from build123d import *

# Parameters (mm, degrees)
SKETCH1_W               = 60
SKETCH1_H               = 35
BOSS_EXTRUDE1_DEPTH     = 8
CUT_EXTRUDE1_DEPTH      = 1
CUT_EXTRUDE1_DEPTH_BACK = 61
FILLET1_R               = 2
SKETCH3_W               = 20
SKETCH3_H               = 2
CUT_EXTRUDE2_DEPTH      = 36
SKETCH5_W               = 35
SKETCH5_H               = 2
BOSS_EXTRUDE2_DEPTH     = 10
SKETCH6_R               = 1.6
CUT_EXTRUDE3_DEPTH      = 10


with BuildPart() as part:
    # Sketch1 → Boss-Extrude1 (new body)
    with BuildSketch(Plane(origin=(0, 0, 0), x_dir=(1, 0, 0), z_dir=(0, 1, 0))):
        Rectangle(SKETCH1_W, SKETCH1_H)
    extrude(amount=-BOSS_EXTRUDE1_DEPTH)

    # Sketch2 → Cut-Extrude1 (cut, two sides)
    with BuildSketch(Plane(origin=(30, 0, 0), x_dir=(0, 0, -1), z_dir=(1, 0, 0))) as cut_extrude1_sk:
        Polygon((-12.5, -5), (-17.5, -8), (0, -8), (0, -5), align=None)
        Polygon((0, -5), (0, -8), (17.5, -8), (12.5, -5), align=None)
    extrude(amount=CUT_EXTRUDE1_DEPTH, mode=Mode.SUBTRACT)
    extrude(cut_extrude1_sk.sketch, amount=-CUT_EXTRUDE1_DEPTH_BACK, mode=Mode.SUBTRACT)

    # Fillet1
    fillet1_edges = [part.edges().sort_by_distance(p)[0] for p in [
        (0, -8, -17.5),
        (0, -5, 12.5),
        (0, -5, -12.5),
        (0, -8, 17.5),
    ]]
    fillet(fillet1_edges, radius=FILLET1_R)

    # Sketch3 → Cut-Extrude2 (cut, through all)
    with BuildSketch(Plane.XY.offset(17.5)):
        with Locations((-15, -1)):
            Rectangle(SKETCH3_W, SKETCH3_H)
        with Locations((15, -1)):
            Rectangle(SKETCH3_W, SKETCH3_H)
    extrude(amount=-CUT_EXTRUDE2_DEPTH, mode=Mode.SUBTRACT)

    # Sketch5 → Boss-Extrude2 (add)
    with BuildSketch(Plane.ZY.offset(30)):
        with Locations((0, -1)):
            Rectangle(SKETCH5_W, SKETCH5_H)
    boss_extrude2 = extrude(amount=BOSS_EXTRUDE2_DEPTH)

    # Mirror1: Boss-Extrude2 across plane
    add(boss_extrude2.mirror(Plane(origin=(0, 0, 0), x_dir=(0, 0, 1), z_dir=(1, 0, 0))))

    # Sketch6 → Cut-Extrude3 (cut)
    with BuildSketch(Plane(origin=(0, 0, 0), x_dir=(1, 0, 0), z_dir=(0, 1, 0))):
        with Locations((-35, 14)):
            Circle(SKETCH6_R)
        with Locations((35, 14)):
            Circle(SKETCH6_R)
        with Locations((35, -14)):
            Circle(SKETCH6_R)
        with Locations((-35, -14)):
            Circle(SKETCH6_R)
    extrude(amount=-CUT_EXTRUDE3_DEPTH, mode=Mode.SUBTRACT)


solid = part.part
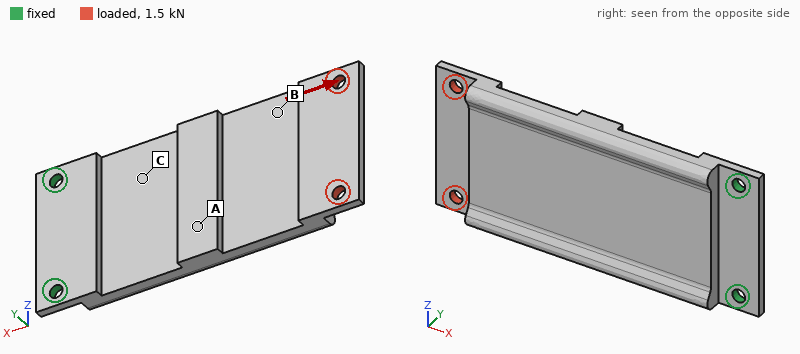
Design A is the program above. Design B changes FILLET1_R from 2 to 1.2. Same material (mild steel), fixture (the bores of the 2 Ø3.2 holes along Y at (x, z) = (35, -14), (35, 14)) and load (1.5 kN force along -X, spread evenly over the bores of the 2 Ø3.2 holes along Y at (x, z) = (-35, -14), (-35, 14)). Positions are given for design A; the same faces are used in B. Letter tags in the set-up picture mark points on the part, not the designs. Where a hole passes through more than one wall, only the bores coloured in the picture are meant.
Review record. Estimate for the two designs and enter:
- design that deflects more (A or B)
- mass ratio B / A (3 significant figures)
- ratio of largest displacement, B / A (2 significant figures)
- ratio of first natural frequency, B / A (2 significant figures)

A
1.02
0.87
1.0
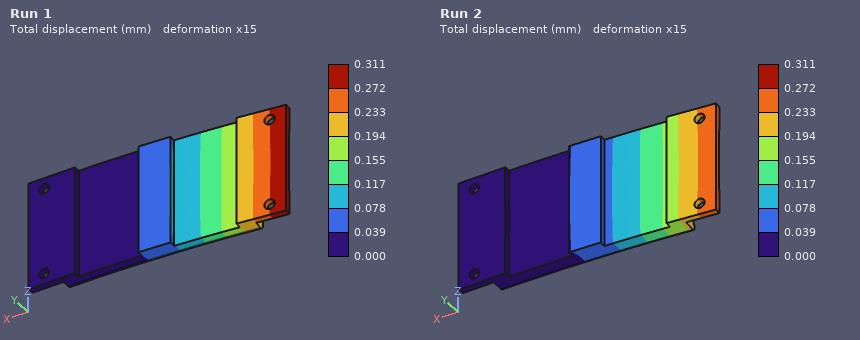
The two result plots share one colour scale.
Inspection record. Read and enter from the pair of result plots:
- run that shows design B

Run 2
